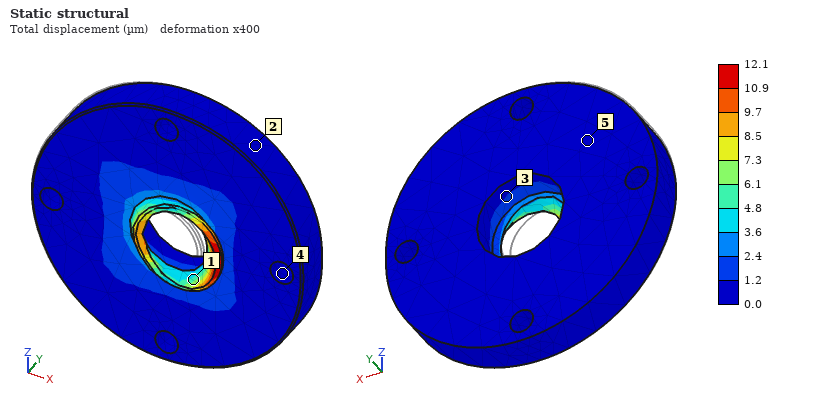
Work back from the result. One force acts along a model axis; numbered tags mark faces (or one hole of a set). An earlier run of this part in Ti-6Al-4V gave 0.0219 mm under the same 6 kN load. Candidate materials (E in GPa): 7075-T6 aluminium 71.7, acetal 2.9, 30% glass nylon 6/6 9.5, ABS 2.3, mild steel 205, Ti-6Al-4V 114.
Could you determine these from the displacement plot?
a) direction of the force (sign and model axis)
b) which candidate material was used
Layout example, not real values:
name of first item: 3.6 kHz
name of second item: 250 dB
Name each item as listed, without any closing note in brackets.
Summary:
direction of the force: +X
which candidate material was used: mild steel
